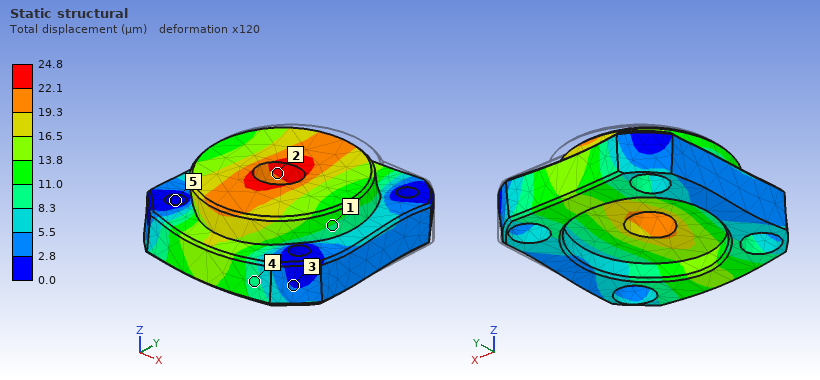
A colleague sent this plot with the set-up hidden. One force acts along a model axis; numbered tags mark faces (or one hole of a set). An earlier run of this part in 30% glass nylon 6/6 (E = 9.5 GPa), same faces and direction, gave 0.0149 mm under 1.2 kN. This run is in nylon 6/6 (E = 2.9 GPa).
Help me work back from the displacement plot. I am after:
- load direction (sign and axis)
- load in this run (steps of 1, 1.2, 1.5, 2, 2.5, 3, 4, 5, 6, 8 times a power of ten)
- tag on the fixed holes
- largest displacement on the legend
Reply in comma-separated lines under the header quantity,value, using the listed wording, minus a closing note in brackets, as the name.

quantity,value
load direction,-Y
load in this run,600 N
tag on the fixed holes,5
largest displacement on the legend,24.8 µm
